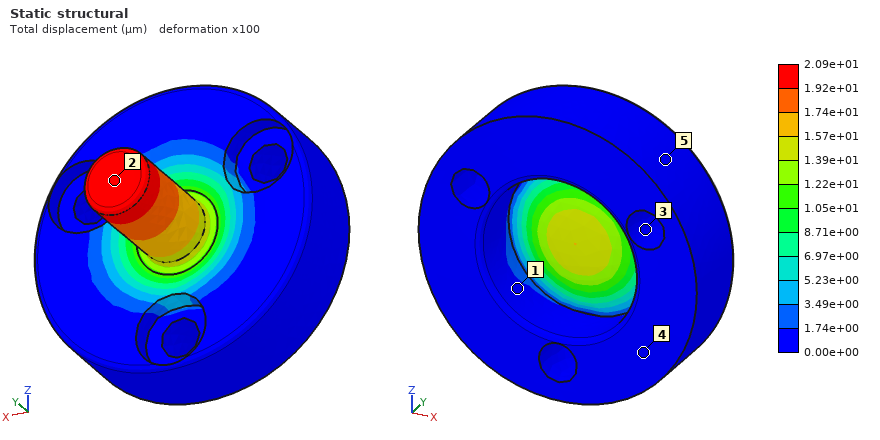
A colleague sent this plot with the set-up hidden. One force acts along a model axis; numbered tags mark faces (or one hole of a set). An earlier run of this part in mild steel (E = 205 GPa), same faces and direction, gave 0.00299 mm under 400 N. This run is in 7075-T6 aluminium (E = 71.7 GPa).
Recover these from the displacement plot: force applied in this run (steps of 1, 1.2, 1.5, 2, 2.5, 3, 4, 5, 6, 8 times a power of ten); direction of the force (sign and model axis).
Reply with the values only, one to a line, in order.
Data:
1 kN
-Y
